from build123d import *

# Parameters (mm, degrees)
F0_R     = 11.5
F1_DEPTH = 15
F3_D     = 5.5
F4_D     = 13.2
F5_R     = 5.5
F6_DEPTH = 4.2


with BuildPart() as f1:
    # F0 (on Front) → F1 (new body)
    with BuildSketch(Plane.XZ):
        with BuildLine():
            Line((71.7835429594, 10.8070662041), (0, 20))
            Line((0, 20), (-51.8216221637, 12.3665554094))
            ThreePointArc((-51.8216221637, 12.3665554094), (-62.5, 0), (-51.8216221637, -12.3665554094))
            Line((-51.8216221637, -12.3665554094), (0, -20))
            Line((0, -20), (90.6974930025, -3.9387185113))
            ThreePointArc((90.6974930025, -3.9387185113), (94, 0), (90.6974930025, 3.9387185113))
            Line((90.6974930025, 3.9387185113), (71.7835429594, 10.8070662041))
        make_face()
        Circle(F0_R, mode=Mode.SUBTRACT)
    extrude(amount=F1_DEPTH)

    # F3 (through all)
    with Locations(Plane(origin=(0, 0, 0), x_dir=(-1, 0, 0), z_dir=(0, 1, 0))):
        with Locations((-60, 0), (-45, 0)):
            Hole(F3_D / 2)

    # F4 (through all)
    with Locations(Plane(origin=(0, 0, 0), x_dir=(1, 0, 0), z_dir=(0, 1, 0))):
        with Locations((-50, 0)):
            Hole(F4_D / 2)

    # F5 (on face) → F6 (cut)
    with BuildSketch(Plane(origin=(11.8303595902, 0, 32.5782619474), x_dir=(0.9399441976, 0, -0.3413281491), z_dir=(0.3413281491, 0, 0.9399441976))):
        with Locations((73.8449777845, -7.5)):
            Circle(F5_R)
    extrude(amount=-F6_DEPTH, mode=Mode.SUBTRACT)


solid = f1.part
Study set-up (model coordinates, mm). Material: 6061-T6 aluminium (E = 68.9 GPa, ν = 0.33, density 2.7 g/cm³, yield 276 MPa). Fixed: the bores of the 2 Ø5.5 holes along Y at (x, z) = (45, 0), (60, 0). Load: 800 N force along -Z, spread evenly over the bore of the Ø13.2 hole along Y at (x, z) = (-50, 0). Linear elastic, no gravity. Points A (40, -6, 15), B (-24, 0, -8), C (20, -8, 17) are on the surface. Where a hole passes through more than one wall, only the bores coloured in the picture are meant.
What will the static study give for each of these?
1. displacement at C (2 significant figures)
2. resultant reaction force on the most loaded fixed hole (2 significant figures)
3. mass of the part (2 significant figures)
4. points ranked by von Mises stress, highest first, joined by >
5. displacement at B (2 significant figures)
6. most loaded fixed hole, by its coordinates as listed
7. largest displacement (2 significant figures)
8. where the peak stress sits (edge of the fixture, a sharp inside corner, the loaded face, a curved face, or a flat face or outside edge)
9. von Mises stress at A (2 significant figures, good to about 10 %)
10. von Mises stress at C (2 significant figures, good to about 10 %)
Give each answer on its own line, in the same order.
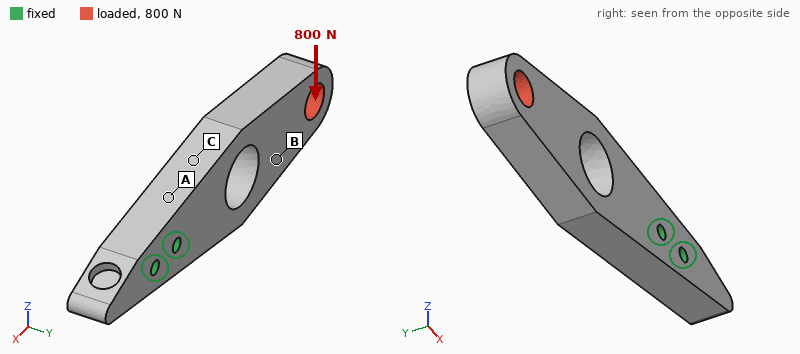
0.037 mm
4.0 kN
150 g
A > C > B
0.12 mm
(45, 0)
0.20 mm
edge of the fixture
38 MPa
25 MPa
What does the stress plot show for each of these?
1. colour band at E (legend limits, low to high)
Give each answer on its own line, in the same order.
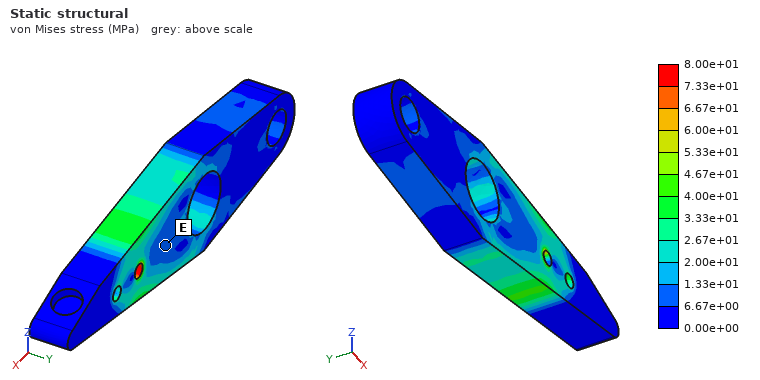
6.67e+00 to 1.33e+01 MPa
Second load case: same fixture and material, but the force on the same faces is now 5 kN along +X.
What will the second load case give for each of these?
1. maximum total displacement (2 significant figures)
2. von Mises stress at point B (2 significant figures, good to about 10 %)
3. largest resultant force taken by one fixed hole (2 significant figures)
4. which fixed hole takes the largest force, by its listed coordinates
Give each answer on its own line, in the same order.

31 µm
10 MPa
3.9 kN
(45, 0)
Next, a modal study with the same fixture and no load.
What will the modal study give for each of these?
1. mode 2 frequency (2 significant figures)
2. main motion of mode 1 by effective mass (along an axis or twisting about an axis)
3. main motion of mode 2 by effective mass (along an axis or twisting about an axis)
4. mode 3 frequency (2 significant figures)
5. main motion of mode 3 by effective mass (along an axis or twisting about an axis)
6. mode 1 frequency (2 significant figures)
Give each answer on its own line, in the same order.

1700 Hz
along Y
along Z
4900 Hz
twisting about X
1100 Hz
